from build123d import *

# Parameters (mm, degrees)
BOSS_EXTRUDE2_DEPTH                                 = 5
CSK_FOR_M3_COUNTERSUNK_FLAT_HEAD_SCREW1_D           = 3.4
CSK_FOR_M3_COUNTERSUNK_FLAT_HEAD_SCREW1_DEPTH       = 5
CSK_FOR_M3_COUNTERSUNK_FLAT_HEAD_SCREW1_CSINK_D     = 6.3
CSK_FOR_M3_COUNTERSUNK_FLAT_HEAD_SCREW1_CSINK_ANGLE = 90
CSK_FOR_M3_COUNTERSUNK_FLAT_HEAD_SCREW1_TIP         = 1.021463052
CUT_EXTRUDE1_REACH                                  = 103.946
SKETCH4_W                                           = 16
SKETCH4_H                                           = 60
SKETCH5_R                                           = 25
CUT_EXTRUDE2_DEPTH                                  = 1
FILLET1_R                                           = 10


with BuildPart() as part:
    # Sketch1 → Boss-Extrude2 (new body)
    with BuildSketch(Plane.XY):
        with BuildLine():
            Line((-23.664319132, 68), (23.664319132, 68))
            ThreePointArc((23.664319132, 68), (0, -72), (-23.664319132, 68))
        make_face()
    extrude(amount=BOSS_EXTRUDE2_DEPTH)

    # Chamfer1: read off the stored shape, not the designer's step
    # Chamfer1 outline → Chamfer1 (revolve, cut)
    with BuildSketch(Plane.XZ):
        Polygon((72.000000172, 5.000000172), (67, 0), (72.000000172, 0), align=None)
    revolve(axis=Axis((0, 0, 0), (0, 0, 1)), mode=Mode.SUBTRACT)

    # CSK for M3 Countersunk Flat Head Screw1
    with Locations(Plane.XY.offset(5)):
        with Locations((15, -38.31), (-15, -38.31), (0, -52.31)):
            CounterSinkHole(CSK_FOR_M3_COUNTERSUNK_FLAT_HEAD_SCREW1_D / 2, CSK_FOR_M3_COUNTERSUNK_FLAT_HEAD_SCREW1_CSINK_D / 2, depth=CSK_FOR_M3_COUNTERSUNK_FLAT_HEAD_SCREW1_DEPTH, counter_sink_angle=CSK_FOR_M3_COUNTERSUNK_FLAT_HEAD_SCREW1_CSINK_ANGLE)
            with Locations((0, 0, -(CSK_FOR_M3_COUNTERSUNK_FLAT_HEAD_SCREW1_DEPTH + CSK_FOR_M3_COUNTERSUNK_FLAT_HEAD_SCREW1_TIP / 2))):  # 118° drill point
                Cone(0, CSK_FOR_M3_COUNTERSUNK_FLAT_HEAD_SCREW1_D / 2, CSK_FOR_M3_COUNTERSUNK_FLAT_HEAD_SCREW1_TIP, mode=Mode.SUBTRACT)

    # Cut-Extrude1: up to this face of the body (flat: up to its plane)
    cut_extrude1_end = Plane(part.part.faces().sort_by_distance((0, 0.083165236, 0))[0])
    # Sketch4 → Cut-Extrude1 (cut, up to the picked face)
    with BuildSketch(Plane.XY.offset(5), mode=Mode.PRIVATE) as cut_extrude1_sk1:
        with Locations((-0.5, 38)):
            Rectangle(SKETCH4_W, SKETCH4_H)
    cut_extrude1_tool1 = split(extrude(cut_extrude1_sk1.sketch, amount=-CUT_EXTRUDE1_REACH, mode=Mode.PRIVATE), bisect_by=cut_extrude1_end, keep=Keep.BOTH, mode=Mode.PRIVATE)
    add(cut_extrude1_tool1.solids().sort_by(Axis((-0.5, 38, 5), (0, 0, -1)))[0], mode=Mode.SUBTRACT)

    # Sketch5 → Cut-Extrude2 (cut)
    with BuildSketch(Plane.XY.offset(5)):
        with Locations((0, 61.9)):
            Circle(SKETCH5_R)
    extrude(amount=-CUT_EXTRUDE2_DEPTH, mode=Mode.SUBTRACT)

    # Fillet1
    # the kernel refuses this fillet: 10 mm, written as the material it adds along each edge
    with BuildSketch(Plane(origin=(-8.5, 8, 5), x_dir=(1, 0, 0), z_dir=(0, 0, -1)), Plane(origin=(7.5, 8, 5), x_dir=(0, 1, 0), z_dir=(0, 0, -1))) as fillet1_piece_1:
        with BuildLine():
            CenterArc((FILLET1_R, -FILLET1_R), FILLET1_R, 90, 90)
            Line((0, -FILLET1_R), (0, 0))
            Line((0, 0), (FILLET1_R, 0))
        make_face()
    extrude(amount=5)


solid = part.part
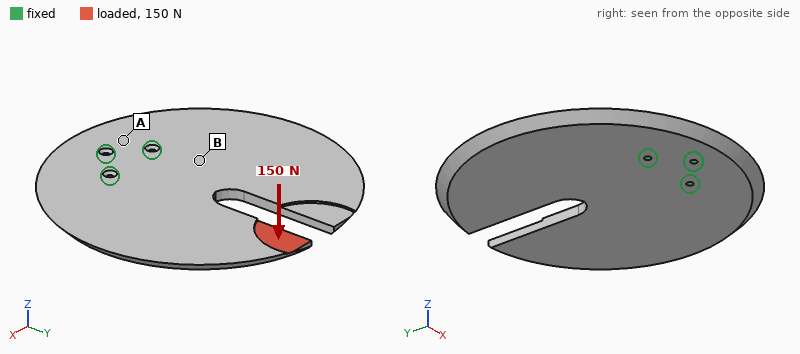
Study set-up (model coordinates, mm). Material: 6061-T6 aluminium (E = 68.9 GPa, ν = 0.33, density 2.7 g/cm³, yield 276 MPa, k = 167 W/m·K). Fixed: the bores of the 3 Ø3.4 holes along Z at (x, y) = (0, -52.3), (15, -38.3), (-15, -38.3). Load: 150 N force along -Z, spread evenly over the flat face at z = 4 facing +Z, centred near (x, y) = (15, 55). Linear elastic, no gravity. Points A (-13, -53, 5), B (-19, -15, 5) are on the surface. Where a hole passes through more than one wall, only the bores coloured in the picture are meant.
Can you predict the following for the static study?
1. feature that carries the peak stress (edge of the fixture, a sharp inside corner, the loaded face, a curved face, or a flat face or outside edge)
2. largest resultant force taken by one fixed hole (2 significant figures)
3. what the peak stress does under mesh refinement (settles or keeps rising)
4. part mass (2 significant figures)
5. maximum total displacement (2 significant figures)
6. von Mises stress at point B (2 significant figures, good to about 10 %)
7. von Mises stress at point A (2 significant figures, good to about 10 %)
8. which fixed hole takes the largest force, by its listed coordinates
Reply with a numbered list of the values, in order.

1. edge of the fixture
2. 400 N
3. keeps rising
4. 190 g
5. 1.1 mm
6. 19 MPa
7. 9.2 MPa
8. (0, -52.3)
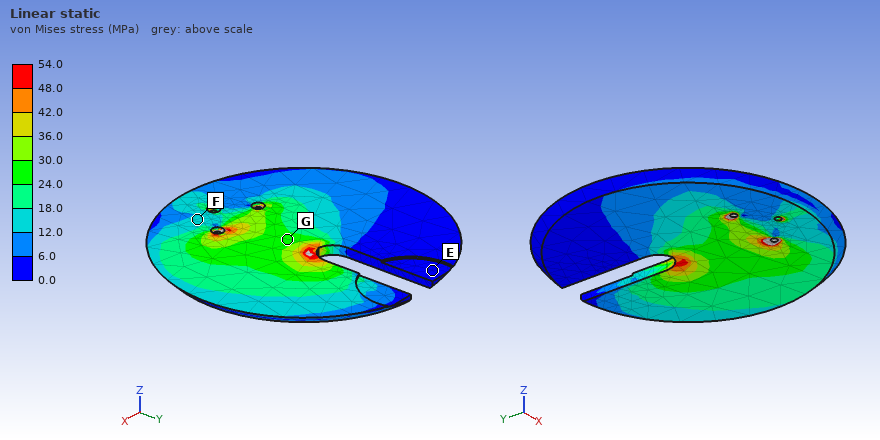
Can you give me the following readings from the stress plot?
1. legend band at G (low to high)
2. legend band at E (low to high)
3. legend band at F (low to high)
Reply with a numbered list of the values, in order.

1. 24.0 to 30.0 MPa
2. 0.0 to 6.0 MPa
3. 12.0 to 18.0 MPa
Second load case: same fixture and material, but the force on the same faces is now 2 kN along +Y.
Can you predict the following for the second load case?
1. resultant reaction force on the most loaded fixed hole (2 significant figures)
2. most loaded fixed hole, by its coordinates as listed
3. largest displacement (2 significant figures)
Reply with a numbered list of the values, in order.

1. 1.6 kN
2. (15, -38.3)
3. 0.45 mm
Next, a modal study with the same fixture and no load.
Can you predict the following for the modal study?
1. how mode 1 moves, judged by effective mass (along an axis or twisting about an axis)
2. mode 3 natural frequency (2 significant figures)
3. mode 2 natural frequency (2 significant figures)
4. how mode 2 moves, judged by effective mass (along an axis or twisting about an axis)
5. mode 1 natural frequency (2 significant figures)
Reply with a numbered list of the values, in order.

1. along Z
2. 1200 Hz
3. 540 Hz
4. twisting about Y
5. 390 Hz
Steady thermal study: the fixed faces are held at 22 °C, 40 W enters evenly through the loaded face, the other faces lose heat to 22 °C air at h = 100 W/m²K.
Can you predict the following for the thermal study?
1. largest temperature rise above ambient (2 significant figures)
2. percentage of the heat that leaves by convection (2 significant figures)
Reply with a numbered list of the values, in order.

1. 68 K
2. 71 %
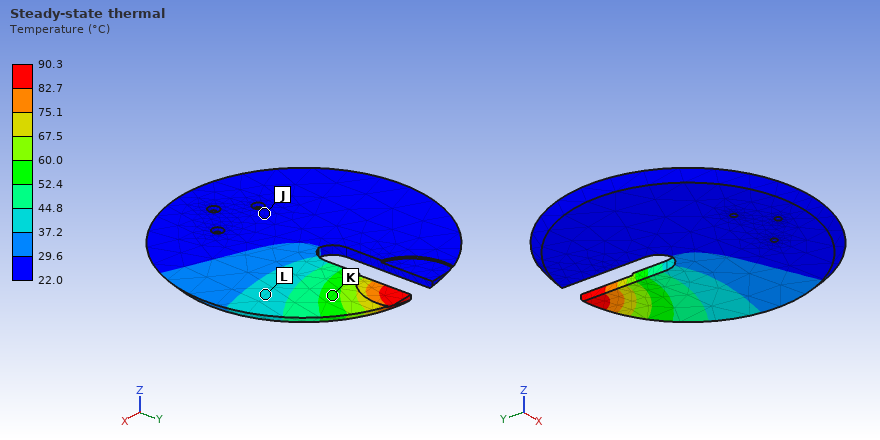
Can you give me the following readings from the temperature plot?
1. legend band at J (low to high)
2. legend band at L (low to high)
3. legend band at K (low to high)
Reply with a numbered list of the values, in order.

1. 22.0 to 29.6 °C
2. 37.2 to 44.8 °C
3. 52.4 to 60.0 °C
